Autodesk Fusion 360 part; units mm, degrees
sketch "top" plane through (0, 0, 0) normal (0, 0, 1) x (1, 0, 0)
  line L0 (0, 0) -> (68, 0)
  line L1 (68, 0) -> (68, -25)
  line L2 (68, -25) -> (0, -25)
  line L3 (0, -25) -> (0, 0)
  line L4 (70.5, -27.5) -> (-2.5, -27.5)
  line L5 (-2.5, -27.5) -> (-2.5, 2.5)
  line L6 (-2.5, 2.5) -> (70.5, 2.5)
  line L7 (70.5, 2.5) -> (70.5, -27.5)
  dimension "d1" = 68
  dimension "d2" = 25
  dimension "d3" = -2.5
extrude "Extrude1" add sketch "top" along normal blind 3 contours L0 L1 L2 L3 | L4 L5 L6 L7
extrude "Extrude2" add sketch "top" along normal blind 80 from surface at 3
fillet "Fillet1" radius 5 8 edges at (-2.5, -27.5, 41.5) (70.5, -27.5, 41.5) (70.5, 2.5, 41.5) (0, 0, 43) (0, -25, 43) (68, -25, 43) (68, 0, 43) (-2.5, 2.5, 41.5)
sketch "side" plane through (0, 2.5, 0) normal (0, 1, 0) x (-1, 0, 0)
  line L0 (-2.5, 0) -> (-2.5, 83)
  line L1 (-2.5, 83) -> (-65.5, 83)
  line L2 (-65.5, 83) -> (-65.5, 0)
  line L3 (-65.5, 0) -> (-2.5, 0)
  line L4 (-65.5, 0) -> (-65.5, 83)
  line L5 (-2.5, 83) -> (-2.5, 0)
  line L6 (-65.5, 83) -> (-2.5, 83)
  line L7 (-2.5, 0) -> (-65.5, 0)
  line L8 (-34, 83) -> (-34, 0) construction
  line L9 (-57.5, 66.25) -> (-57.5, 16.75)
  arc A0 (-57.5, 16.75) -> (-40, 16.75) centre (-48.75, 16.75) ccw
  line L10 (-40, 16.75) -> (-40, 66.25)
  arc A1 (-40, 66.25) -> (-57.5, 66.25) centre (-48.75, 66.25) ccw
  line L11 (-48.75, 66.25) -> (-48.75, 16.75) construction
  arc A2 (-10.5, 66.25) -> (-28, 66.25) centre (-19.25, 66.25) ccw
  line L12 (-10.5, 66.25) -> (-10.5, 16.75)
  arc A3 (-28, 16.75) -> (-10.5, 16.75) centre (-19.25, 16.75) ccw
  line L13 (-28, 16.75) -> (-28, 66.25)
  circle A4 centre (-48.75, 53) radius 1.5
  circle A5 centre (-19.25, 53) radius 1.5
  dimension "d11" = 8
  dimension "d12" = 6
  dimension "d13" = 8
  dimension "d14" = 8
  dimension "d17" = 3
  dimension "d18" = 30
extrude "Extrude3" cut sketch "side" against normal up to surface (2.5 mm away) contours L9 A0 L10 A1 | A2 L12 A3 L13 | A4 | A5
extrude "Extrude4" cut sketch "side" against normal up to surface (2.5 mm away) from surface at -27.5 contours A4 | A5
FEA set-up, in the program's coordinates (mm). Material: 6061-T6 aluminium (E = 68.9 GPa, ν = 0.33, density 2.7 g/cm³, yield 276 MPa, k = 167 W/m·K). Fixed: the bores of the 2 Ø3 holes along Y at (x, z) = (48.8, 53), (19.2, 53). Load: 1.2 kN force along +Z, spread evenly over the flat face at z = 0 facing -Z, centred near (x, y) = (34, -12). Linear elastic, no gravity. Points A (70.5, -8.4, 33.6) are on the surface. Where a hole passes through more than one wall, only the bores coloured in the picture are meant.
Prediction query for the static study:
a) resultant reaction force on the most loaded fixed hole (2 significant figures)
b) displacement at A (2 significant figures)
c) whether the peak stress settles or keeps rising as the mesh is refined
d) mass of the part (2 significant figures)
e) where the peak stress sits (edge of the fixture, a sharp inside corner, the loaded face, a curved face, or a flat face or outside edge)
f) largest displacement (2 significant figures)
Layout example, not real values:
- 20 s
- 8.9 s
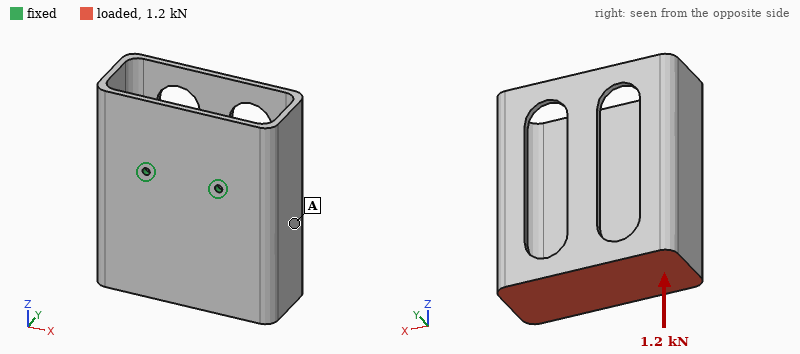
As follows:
- 600 N
- 0.53 mm
- keeps rising
- 110 g
- edge of the fixture
- 1.2 mm
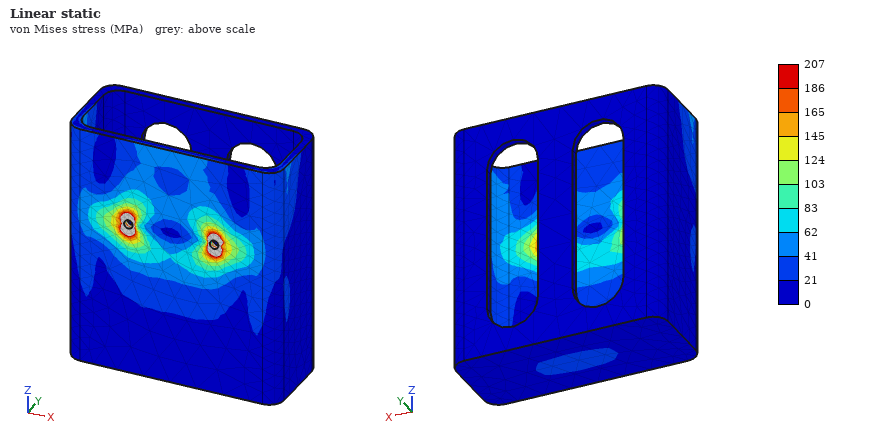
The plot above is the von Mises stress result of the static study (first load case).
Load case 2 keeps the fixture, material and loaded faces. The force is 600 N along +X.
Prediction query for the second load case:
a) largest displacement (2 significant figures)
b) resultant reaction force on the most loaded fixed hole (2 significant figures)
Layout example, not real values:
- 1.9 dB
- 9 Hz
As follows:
- 0.23 mm
- 1.1 kN
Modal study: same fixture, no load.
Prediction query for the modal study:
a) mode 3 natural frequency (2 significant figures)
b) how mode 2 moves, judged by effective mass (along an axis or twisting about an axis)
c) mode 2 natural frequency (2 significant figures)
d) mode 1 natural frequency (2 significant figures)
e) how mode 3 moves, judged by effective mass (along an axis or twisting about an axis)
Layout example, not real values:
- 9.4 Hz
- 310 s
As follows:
- 1400 Hz
- along X
- 720 Hz
- 390 Hz
- along Y
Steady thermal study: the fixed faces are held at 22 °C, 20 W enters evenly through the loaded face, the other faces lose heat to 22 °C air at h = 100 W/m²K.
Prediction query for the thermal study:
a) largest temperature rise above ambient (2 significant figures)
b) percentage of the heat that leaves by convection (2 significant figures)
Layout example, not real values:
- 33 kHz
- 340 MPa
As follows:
- 13 K
- 75 %
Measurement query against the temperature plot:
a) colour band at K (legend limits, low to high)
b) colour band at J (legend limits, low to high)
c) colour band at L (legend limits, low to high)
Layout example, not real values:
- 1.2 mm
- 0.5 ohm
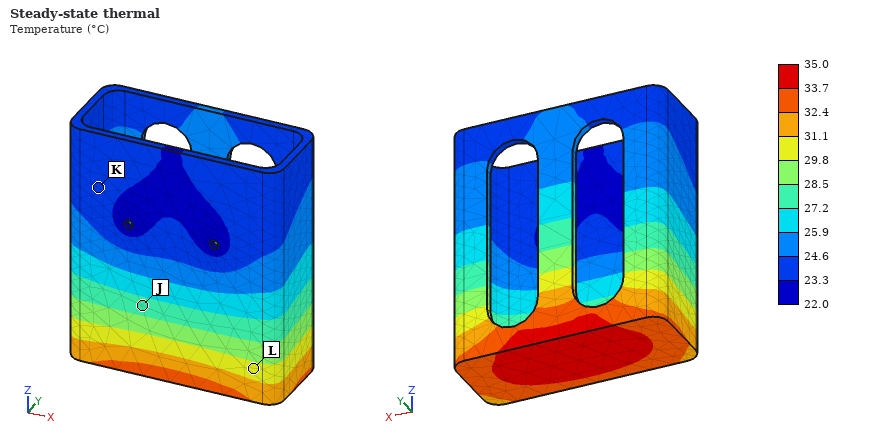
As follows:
- 23.3 to 24.6 °C
- 27.2 to 28.5 °C
- 29.8 to 31.1 °C
